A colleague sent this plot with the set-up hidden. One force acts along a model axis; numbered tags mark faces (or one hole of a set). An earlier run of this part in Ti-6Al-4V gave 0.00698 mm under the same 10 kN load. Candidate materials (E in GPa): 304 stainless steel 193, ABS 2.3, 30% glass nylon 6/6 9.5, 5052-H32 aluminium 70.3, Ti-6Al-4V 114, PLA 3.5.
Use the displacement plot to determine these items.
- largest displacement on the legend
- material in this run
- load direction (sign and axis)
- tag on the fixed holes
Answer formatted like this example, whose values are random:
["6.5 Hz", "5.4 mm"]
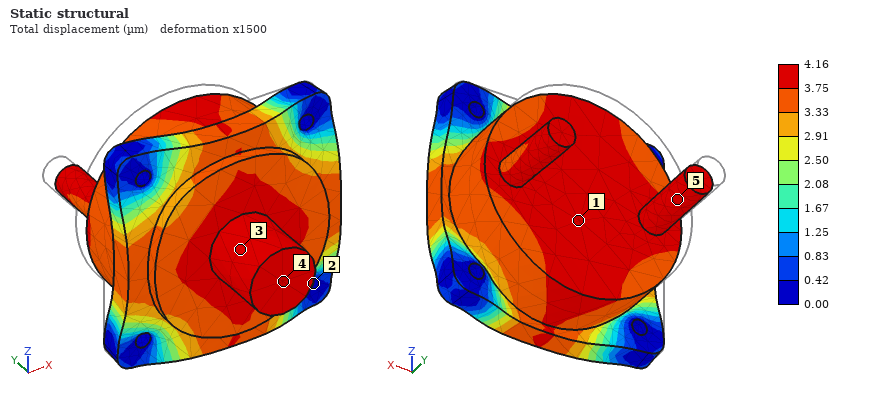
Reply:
["4.16 µm", "304 stainless steel", "-Y", "2"]
